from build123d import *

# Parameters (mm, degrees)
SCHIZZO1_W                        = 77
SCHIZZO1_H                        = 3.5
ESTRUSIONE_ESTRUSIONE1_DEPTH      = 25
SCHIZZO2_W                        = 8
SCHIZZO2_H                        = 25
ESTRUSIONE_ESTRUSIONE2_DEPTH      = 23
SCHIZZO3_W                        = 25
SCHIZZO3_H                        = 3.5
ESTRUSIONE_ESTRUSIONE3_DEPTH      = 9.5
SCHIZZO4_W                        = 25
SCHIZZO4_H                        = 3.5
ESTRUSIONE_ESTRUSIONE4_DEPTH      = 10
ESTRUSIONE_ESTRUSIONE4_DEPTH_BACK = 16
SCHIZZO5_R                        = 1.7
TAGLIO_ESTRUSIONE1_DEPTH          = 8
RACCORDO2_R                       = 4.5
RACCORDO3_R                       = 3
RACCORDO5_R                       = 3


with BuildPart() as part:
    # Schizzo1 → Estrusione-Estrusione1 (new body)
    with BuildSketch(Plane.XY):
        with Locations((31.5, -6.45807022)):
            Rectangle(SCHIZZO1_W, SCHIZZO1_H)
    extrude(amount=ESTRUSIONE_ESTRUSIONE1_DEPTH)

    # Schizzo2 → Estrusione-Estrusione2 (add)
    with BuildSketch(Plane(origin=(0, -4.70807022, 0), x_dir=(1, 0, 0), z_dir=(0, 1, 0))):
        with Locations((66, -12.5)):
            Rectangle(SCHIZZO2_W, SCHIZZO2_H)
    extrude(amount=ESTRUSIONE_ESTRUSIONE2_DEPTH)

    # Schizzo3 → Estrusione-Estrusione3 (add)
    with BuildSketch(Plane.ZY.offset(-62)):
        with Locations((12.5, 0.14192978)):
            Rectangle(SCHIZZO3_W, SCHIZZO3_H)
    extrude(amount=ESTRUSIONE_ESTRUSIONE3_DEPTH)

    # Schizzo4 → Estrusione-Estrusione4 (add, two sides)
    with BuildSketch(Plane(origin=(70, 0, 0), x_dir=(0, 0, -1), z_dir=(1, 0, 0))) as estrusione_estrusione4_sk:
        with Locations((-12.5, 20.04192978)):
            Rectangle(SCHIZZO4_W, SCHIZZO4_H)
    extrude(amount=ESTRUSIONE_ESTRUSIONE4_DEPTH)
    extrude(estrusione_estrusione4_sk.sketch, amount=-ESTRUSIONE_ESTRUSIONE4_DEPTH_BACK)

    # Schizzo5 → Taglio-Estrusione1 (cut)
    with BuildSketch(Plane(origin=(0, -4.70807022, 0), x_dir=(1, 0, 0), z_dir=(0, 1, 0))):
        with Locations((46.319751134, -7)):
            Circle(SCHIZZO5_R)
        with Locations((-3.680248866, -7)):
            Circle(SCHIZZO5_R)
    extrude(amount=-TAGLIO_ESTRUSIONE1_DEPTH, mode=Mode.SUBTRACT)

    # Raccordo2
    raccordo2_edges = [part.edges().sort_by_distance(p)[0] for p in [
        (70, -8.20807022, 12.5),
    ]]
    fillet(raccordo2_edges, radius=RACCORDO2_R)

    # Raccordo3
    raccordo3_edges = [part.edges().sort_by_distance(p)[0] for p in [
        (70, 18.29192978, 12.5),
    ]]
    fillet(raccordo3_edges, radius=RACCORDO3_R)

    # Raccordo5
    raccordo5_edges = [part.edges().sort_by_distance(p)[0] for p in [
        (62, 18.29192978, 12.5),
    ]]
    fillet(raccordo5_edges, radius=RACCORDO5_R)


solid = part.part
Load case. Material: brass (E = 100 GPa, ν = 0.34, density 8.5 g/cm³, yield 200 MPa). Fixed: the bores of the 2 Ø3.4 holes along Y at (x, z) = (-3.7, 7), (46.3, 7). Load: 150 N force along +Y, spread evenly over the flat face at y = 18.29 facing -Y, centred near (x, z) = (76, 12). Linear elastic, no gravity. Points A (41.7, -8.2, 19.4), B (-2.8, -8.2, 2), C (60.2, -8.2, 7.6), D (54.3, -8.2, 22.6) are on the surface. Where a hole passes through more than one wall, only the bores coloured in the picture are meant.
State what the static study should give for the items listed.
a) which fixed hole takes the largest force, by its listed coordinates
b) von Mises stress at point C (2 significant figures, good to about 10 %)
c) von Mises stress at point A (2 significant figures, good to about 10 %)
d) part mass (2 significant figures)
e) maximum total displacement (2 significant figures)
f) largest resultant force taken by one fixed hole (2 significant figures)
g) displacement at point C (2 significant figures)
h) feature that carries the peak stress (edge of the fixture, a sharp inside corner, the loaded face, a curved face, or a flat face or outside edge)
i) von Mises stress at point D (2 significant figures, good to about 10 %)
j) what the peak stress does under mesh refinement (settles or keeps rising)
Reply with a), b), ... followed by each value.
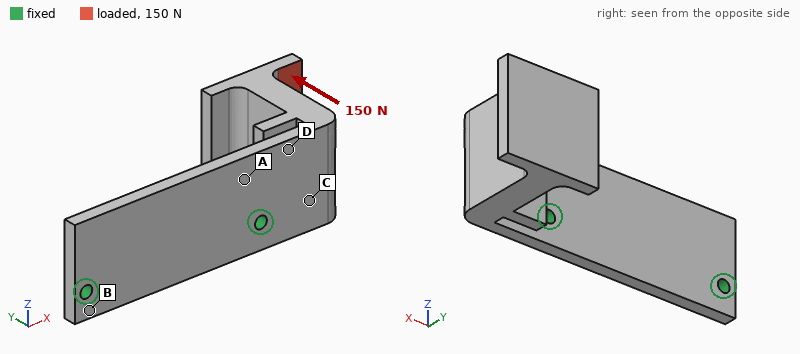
a) (46.3, 7)
b) 44 MPa
c) 30 MPa
d) 120 g
e) 0.29 mm
f) 170 N
g) 0.050 mm
h) edge of the fixture
i) 52 MPa
j) keeps rising
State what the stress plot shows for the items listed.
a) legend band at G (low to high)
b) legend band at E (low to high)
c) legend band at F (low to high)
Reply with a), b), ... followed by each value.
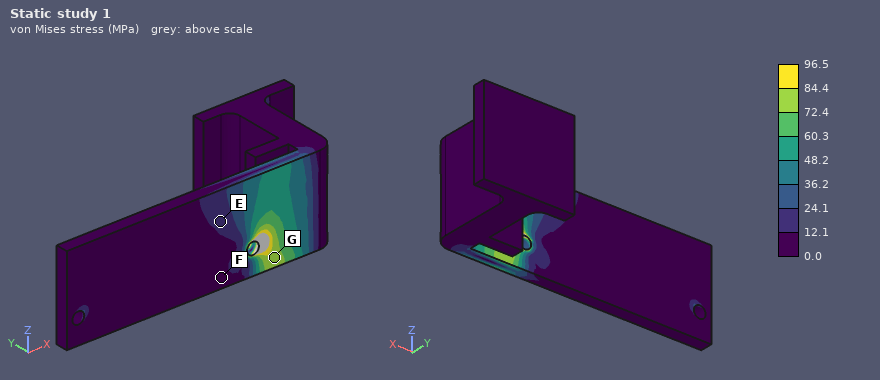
a) 72.4 to 84.4 MPa
b) 12.1 to 24.1 MPa
c) 0.0 to 12.1 MPa
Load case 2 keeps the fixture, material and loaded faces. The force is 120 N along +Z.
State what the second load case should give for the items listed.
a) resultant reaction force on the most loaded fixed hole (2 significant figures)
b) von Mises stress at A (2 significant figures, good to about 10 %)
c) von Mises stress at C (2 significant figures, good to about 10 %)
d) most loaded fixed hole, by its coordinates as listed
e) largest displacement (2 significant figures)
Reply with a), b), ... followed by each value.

a) 200 N
b) 27 MPa
c) 27 MPa
d) (46.3, 7)
e) 0.12 mm
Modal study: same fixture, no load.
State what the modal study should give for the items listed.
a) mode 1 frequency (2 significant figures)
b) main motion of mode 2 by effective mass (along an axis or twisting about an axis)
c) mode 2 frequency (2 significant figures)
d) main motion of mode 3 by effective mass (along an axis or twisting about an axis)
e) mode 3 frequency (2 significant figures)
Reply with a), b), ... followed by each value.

a) 590 Hz
b) along Z
c) 870 Hz
d) along Y
e) 2500 Hz
